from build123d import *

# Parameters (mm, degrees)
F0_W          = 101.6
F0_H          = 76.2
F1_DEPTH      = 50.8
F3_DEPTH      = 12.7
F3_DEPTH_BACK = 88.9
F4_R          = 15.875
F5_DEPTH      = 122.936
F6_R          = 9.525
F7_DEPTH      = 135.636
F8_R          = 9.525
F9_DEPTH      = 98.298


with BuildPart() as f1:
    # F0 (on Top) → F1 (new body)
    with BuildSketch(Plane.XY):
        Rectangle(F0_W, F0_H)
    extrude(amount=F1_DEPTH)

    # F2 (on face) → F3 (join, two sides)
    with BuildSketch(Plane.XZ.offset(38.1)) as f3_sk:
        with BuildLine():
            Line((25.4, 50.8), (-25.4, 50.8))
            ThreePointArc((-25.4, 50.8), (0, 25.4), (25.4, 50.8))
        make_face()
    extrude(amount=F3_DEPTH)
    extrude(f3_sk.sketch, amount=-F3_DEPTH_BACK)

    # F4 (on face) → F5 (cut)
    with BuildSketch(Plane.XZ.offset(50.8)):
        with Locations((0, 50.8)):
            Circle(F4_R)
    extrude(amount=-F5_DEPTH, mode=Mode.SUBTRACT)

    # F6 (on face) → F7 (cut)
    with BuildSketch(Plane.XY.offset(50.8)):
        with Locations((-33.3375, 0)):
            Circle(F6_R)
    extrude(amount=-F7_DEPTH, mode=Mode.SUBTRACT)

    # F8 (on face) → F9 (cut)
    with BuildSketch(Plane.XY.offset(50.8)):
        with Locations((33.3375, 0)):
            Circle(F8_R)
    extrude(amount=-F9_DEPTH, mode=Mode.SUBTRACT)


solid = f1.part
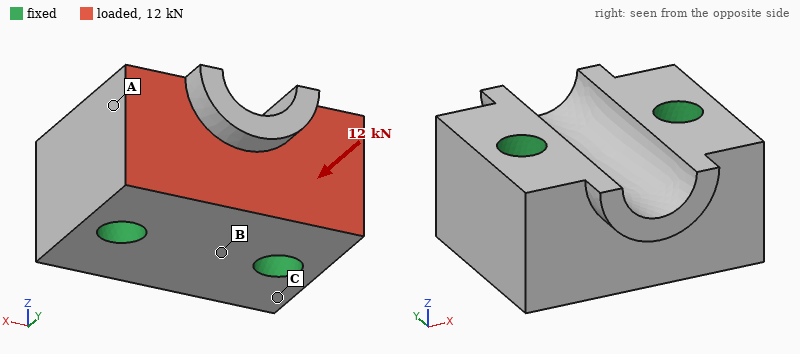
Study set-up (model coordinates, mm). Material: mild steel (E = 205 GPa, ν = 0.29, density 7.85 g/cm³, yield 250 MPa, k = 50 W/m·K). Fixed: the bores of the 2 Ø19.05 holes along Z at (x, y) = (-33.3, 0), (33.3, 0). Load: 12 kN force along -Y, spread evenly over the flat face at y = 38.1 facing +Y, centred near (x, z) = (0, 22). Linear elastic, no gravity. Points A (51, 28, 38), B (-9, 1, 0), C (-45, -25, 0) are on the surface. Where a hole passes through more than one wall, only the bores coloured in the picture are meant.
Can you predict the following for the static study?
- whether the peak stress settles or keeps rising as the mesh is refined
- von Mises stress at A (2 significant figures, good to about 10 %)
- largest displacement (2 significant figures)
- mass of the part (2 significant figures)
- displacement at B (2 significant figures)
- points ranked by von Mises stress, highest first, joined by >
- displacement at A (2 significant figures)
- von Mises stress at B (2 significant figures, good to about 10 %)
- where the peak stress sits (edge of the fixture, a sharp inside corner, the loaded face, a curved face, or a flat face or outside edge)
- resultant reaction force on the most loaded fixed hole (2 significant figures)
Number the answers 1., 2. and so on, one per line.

1. keeps rising
2. 2.8 MPa
3. 0.72 µm
4. 2.7 kg
5. 0.26 µm
6. A > B > C
7. 0.36 µm
8. 1.4 MPa
9. edge of the fixture
10. 6.0 kN
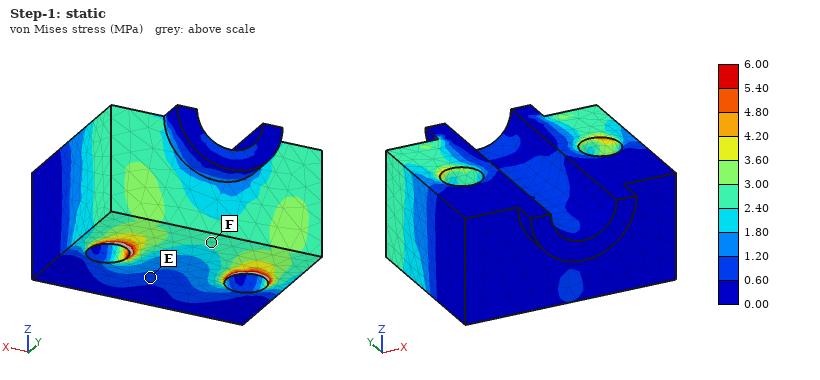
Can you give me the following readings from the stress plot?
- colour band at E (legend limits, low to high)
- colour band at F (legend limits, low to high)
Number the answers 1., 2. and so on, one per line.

1. 0.60 to 1.20 MPa
2. 2.40 to 3.00 MPa
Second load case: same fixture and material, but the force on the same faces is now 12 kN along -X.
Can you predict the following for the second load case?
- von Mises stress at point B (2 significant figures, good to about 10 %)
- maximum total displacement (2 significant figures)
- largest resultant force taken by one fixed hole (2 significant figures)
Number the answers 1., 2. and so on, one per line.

1. 2.4 MPa
2. 2.4 µm
3. 7.6 kN
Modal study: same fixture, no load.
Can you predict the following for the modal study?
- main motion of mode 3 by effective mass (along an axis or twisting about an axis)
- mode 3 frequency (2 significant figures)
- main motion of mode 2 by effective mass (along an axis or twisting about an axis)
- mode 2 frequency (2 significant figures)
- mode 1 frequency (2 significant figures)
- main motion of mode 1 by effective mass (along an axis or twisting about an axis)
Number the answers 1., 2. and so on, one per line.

1. twisting about Z
2. 17 kHz
3. along Z
4. 16 kHz
5. 15 kHz
6. twisting about X
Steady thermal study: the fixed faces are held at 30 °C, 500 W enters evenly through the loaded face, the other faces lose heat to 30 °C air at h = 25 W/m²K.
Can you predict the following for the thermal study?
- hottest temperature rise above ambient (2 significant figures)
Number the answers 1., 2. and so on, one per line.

1. 78 K
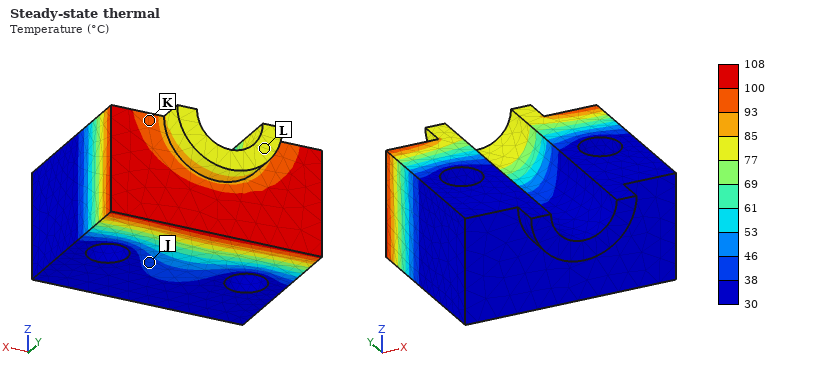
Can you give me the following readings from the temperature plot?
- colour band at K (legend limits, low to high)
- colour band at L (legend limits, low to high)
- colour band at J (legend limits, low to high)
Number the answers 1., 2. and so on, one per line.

1. 93 to 100 °C
2. 77 to 85 °C
3. 38 to 46 °C
